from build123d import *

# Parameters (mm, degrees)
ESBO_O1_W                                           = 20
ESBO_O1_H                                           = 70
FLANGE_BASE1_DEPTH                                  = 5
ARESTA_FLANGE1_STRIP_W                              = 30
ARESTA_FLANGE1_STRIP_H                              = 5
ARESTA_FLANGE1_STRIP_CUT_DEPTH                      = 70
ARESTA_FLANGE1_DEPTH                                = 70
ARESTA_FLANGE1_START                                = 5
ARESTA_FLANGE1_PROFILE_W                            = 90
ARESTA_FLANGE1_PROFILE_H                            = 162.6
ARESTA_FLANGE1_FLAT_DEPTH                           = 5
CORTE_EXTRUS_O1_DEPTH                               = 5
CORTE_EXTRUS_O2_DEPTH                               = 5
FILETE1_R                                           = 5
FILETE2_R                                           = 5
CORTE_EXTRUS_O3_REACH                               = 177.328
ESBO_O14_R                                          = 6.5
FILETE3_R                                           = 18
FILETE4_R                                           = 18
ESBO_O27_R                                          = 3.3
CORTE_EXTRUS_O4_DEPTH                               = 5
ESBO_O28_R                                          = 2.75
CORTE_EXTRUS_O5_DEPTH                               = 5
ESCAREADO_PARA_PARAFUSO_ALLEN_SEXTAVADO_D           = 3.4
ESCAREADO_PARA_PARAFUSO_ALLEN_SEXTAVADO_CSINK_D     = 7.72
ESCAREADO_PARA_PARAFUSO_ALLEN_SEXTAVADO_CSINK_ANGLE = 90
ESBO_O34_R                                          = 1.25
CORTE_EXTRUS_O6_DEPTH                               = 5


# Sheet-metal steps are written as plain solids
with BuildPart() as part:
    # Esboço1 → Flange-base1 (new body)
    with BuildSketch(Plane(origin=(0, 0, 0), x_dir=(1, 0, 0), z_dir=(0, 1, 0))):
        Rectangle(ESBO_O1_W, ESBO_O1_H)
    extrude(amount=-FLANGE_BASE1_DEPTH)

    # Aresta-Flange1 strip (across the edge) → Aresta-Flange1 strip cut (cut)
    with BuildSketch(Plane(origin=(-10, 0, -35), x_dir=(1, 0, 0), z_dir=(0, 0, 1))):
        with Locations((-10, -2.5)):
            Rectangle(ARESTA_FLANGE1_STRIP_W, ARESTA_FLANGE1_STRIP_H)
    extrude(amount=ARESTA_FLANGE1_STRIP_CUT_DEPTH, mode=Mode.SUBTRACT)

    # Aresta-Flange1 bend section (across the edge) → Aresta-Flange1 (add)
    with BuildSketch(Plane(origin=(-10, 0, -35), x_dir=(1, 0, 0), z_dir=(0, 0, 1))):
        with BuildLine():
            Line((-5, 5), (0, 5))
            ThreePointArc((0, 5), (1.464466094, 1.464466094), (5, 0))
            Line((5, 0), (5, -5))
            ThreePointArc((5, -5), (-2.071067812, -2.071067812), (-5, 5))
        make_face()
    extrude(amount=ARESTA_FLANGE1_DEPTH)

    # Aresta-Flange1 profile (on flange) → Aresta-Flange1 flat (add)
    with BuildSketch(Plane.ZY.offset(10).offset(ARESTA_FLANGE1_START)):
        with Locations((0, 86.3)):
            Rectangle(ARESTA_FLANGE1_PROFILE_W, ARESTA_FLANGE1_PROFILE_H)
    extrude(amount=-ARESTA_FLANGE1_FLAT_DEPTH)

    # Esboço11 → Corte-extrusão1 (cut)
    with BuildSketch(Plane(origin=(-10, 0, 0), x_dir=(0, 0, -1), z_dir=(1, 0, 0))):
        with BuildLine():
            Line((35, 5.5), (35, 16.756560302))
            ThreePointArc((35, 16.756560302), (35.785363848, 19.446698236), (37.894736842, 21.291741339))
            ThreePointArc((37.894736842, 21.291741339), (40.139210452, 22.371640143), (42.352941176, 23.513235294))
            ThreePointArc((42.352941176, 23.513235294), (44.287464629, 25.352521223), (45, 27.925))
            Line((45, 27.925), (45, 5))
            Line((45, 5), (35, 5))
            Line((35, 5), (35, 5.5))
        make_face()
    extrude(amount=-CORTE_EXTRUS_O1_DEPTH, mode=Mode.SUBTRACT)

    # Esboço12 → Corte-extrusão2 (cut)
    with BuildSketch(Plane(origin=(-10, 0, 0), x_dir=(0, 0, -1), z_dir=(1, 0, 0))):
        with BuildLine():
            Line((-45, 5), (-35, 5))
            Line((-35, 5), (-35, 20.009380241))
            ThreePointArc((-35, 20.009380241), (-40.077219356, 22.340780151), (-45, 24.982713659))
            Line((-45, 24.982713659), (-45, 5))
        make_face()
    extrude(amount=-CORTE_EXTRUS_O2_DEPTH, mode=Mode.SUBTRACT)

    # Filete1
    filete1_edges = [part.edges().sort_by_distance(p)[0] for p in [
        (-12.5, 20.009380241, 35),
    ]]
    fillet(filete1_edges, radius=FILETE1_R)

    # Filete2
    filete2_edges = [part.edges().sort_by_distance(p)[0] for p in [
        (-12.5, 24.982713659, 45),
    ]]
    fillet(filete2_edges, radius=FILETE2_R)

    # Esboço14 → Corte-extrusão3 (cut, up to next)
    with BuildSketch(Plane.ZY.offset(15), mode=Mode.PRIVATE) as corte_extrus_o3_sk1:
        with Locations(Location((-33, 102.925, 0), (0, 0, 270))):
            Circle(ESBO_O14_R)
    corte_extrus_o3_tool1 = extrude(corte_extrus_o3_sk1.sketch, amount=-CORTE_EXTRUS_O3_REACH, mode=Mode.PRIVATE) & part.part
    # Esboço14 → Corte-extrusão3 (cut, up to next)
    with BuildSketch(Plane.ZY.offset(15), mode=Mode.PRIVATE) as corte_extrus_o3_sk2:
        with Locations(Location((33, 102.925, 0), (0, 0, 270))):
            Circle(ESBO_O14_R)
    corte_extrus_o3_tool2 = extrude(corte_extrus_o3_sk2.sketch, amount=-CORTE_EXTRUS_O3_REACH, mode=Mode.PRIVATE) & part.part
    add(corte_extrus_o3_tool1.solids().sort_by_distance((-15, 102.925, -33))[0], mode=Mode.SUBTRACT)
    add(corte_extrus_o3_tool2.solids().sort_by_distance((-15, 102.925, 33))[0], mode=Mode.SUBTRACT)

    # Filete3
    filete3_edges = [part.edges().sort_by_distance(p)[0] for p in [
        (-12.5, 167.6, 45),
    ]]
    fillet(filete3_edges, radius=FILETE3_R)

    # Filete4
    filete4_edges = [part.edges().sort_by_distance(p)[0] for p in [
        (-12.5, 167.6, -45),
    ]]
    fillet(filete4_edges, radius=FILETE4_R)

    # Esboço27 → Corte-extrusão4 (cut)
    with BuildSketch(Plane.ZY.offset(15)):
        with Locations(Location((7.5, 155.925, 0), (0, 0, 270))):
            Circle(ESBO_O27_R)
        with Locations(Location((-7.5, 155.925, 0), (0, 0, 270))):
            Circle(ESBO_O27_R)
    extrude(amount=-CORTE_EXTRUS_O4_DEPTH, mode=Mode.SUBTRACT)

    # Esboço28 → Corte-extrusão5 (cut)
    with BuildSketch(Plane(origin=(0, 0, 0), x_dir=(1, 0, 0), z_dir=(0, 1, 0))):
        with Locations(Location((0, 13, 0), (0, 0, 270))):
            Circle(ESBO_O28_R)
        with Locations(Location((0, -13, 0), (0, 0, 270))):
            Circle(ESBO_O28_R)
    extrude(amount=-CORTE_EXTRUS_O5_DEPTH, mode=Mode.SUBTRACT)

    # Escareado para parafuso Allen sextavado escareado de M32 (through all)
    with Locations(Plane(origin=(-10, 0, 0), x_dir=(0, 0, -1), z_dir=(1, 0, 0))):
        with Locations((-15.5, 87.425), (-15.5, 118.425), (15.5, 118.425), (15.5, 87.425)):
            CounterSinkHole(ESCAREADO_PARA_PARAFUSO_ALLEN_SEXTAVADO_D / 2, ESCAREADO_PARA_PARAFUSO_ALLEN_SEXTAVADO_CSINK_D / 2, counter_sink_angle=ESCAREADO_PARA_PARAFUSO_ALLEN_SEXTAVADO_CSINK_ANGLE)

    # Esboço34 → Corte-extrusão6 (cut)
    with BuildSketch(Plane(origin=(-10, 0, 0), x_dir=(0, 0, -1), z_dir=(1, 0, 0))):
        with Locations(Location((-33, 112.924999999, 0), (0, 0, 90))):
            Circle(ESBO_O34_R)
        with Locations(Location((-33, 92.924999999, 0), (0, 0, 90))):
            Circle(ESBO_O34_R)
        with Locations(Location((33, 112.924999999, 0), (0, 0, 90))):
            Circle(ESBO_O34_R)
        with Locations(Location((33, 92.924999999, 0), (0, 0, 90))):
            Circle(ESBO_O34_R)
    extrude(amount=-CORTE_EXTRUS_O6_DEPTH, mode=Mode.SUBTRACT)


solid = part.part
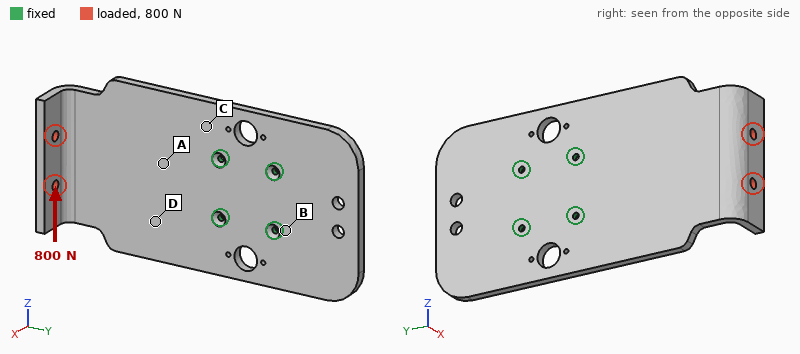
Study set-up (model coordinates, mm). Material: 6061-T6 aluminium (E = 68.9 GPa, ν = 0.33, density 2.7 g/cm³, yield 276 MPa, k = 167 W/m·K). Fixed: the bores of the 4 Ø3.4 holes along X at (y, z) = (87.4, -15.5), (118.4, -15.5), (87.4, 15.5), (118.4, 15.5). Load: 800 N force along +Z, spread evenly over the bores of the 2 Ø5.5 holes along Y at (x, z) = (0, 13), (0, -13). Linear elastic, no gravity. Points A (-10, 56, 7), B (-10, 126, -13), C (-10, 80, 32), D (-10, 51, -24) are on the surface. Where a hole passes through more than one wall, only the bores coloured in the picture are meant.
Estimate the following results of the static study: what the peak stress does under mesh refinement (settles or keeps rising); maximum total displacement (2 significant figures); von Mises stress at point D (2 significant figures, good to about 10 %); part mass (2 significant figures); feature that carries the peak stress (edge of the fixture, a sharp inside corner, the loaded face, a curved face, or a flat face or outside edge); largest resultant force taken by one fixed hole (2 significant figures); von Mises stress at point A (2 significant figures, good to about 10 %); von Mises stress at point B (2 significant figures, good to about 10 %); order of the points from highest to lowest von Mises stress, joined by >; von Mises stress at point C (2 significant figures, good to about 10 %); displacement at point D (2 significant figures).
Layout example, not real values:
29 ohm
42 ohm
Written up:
keeps rising
0.38 mm
22 MPa
210 g
edge of the fixture
1.4 kN
29 MPa
4.0 MPa
A > D > C > B
12 MPa
0.082 mm
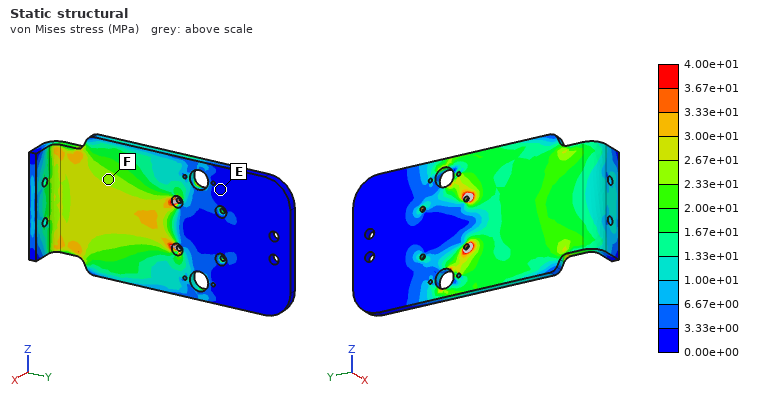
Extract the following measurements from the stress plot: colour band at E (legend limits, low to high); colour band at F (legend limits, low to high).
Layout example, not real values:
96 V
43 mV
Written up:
0.00e+00 to 3.33e+00 MPa
2.33e+01 to 2.67e+01 MPa
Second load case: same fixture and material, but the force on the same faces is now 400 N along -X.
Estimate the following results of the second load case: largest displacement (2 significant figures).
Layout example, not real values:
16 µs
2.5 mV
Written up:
2.0 mm
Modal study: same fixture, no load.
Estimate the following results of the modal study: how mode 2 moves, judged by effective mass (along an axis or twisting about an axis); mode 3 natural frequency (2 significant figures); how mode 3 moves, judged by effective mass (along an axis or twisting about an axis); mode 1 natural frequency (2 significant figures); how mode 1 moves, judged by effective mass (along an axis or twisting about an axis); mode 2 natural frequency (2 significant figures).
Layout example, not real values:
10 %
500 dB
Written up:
twisting about Y
1400 Hz
along X
370 Hz
along X
1000 Hz
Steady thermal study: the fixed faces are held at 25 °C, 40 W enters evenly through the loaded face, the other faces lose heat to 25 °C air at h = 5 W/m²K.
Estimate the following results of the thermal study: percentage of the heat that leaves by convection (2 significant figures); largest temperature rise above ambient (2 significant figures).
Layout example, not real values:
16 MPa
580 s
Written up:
8.4 %
67 K
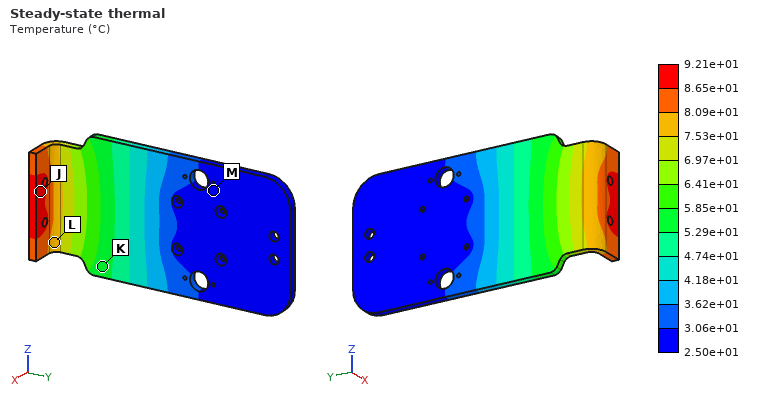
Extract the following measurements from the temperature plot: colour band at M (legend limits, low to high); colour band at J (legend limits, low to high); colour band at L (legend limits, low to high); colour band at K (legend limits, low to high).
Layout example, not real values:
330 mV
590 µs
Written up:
2.50e+01 to 3.06e+01 °C
8.65e+01 to 9.21e+01 °C
7.53e+01 to 8.09e+01 °C
5.29e+01 to 5.85e+01 °C
